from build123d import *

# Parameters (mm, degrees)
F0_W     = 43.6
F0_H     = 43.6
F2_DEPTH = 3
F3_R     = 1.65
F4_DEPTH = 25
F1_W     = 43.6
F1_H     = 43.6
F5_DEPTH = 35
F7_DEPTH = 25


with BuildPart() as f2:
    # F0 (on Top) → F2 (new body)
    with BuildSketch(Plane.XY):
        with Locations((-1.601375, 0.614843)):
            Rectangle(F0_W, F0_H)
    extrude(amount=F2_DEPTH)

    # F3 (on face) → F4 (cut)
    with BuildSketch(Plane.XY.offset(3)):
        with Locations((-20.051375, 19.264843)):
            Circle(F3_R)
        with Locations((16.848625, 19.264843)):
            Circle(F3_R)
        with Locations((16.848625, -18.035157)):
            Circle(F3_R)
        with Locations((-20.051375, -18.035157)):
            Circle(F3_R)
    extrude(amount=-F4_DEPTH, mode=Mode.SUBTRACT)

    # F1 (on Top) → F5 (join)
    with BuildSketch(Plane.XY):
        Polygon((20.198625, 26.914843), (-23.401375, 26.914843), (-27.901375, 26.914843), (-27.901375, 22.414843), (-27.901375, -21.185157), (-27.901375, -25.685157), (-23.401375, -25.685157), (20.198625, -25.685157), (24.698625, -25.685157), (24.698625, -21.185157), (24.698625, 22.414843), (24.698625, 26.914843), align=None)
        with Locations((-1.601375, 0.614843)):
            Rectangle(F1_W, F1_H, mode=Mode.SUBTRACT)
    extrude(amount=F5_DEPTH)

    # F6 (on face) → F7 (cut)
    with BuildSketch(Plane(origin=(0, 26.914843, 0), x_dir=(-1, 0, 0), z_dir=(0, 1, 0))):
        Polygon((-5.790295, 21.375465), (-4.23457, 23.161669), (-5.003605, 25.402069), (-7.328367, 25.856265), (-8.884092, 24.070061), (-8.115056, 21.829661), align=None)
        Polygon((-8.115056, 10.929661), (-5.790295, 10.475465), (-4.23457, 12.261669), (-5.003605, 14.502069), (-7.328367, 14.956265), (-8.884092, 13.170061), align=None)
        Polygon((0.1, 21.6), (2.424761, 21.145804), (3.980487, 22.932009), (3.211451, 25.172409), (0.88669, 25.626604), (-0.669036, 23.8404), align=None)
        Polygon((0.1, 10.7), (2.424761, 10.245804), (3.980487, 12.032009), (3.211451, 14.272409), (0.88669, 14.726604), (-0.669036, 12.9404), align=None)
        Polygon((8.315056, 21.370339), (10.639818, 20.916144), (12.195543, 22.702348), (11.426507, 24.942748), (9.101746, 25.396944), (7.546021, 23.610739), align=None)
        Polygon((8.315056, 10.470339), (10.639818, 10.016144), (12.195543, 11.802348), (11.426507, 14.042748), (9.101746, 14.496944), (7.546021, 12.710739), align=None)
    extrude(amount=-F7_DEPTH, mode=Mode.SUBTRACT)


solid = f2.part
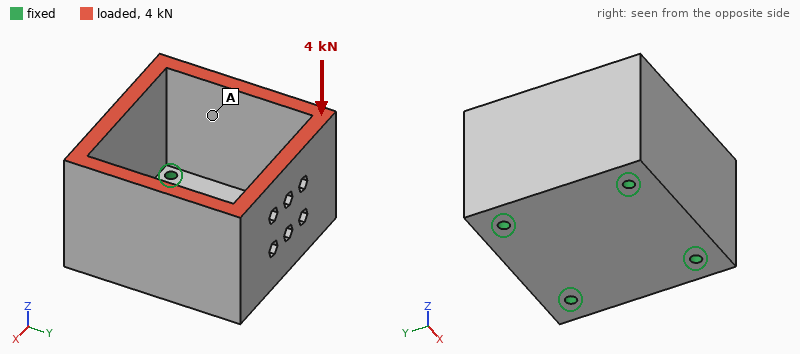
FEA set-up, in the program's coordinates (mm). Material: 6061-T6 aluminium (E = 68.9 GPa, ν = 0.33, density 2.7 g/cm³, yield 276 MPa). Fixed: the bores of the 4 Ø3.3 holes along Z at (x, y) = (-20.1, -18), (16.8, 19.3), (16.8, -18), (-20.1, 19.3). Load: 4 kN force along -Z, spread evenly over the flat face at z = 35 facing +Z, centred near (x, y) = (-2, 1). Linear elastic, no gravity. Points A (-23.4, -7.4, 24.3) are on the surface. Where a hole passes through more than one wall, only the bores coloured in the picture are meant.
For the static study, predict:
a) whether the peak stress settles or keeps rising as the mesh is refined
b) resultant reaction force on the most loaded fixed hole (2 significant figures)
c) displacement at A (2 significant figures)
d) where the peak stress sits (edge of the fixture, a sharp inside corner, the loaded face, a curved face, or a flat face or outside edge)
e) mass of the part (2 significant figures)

keeps rising
1.0 kN
8.4 µm
edge of the fixture
96 g
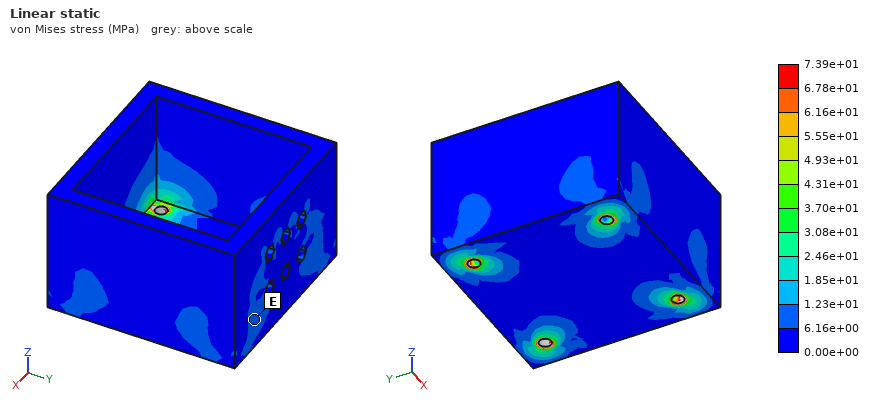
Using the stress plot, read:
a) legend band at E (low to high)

6.16e+00 to 1.23e+01 MPa
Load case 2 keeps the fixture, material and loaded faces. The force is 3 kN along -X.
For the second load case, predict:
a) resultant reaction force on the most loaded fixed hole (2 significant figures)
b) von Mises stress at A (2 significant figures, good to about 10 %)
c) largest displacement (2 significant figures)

1.5 kN
26 MPa
94 µm
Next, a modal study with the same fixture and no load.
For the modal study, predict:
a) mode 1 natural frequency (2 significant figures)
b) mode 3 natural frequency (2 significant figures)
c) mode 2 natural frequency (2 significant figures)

6400 Hz
6800 Hz
6700 Hz
